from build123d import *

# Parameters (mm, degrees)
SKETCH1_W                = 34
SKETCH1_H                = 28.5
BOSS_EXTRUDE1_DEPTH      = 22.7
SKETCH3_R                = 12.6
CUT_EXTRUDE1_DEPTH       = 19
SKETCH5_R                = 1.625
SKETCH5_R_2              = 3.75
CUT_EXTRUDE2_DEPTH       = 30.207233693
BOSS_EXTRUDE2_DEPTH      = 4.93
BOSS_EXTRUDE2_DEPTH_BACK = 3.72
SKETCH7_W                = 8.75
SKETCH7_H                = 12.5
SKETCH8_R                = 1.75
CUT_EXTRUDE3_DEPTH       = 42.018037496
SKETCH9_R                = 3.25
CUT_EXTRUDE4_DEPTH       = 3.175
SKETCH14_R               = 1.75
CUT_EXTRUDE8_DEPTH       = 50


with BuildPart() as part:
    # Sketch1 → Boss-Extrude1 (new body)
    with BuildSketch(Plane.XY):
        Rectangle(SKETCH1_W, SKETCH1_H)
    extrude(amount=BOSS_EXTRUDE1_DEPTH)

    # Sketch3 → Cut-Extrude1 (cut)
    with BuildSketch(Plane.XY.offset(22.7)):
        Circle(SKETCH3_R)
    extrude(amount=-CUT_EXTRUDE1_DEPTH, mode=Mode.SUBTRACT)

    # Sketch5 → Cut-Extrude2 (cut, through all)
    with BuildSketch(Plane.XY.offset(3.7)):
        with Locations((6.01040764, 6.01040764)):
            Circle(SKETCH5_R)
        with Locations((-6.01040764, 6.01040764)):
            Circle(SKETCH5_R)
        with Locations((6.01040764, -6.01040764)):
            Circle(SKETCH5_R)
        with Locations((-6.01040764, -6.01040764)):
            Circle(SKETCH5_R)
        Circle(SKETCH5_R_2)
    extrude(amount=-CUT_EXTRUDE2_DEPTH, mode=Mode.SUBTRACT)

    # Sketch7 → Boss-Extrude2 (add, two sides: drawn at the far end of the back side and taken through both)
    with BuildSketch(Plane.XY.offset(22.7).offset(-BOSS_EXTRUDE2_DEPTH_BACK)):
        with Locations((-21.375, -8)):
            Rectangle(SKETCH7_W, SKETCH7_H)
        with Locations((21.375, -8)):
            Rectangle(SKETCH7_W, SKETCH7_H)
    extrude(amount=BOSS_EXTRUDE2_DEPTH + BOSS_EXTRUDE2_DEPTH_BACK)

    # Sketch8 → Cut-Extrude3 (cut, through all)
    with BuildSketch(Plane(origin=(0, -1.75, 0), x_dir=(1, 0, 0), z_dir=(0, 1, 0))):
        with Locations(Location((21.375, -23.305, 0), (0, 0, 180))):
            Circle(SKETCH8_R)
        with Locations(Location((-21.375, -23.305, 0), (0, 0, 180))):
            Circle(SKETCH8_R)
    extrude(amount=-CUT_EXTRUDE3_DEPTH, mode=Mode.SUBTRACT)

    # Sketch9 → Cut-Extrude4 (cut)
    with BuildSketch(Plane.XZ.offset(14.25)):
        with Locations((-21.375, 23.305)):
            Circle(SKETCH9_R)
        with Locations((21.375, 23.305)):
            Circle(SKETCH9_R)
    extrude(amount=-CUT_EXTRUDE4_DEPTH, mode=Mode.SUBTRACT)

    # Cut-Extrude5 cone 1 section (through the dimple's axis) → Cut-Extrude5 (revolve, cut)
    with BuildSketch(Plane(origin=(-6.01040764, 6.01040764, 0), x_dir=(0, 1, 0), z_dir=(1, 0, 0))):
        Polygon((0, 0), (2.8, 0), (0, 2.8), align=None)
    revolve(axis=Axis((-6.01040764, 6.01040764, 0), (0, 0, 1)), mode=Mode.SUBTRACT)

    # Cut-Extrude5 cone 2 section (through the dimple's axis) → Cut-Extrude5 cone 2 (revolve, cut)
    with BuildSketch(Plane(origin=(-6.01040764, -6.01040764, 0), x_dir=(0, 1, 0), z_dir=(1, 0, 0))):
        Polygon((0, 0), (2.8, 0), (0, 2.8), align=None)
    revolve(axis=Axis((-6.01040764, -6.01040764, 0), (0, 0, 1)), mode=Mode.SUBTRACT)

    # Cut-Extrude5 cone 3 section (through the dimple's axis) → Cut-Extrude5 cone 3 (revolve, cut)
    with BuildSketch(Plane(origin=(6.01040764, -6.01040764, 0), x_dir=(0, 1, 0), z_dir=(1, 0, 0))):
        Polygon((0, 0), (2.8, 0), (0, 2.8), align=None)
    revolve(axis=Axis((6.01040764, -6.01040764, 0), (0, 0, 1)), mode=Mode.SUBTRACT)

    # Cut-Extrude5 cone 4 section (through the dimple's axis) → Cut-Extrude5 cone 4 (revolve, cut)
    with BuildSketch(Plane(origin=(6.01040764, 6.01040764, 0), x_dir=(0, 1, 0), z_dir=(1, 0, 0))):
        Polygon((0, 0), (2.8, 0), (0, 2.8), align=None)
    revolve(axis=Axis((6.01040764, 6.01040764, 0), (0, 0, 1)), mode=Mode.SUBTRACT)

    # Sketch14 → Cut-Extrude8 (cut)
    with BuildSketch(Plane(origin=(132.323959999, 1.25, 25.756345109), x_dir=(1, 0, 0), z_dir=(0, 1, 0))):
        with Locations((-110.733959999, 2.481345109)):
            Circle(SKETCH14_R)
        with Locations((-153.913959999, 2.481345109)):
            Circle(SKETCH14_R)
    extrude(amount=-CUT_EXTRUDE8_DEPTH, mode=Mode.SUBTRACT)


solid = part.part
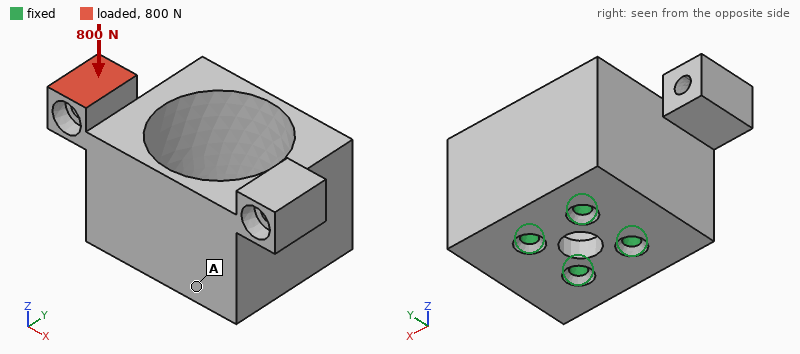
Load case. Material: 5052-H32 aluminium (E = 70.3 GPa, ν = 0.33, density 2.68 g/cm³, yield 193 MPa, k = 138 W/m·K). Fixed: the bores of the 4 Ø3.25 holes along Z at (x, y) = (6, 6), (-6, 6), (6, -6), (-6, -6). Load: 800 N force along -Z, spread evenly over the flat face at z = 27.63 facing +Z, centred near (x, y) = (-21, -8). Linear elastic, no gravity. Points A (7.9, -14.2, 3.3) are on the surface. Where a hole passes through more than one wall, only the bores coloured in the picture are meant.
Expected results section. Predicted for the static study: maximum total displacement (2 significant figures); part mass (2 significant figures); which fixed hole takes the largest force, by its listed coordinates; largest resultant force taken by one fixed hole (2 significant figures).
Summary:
0.11 mm
37 g
(-6, -6)
1.0 kN
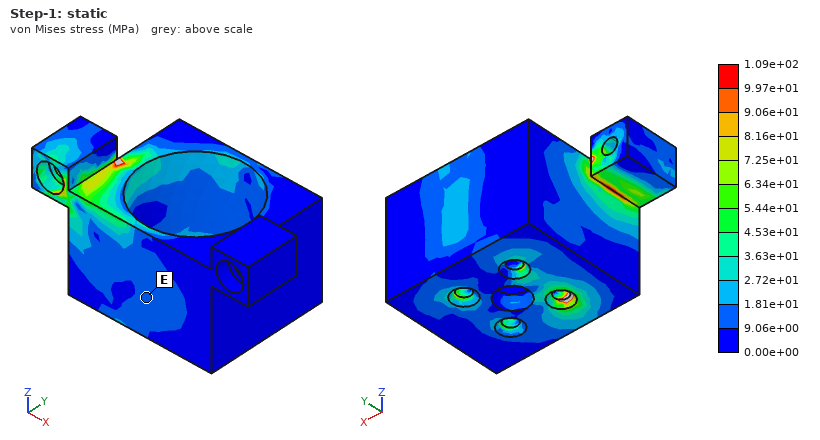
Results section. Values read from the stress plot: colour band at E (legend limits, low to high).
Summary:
9.06e+00 to 1.81e+01 MPa
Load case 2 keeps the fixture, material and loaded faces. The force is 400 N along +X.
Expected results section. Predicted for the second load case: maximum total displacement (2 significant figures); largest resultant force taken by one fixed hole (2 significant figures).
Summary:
78 µm
390 N
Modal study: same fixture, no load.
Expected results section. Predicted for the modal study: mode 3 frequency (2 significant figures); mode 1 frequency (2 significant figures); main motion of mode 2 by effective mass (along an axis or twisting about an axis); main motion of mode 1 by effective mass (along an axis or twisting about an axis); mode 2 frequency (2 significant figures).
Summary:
10 kHz
6000 Hz
along Y
along X
7300 Hz
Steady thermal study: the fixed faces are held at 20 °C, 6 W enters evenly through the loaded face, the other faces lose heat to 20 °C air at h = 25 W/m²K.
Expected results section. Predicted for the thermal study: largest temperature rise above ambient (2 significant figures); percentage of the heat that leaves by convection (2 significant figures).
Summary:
15 K
7.2 %
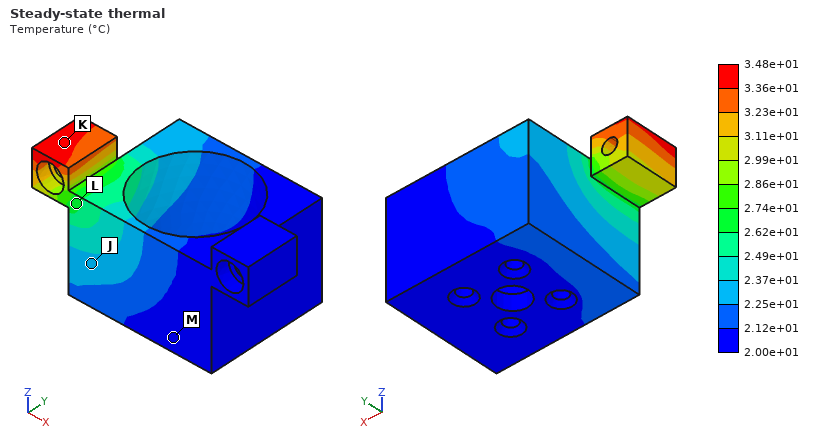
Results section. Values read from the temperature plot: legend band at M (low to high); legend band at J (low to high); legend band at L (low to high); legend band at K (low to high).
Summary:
2.00e+01 to 2.12e+01 °C
2.25e+01 to 2.37e+01 °C
2.62e+01 to 2.74e+01 °C
3.36e+01 to 3.48e+01 °C
